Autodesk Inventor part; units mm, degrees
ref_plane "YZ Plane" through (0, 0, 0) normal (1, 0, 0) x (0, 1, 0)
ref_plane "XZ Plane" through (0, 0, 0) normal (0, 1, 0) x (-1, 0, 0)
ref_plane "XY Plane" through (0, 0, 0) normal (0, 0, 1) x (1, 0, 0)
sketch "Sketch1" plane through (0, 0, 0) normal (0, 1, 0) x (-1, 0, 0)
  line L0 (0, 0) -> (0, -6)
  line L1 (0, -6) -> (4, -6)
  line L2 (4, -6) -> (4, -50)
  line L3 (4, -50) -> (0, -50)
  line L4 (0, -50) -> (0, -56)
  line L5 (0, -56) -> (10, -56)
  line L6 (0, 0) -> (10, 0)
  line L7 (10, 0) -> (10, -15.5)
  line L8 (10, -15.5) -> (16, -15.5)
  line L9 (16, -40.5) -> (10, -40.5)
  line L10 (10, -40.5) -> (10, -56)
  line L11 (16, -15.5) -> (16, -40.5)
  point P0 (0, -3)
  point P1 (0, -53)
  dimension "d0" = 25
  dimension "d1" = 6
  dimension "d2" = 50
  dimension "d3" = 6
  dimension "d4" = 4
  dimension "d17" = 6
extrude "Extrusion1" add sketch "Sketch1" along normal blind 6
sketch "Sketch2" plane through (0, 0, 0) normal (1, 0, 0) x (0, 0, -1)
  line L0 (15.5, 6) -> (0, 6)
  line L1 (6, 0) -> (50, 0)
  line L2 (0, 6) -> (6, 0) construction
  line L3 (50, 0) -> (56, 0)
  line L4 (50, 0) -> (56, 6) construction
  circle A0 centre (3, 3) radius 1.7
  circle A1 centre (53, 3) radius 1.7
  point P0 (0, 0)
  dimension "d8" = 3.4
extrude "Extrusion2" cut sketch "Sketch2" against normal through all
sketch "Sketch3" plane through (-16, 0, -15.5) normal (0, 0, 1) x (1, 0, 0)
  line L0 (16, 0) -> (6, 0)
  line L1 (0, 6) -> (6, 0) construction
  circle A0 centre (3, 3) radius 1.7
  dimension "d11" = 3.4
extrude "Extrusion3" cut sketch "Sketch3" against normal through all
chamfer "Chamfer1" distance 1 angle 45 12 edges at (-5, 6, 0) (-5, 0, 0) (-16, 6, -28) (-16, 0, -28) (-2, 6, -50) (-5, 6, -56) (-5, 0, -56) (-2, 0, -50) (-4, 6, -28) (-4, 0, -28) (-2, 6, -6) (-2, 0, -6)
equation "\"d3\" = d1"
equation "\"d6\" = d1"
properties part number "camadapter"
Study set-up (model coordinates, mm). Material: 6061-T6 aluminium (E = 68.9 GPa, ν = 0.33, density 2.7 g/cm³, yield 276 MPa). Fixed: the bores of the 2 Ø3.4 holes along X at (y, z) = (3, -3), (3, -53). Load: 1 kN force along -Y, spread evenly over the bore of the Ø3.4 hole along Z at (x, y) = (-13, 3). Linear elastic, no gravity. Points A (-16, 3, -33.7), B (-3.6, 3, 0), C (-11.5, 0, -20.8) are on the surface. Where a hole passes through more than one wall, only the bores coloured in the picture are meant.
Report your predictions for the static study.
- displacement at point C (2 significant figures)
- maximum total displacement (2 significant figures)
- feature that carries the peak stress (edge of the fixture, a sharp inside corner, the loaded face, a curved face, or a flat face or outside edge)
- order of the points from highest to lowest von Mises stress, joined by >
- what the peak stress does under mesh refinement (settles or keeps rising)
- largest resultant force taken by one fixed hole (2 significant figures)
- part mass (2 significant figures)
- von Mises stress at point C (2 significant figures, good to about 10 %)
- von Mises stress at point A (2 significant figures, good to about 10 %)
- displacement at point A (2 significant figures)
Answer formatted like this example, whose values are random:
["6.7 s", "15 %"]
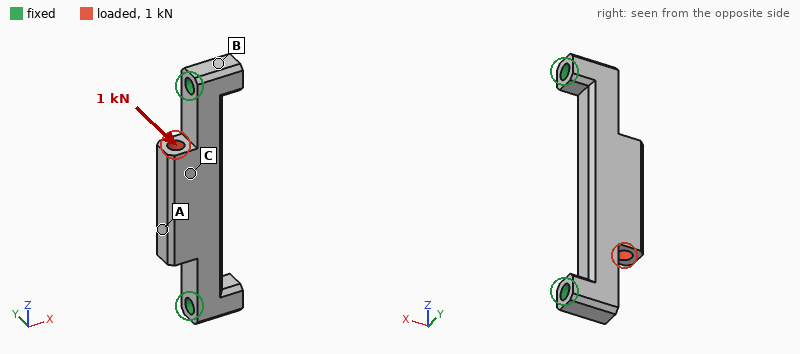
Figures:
["0.099 mm", "0.15 mm", "edge of the fixture", "C > A > B", "keeps rising", "500 N", "7.3 g", "60 MPa", "30 MPa", "0.14 mm"]
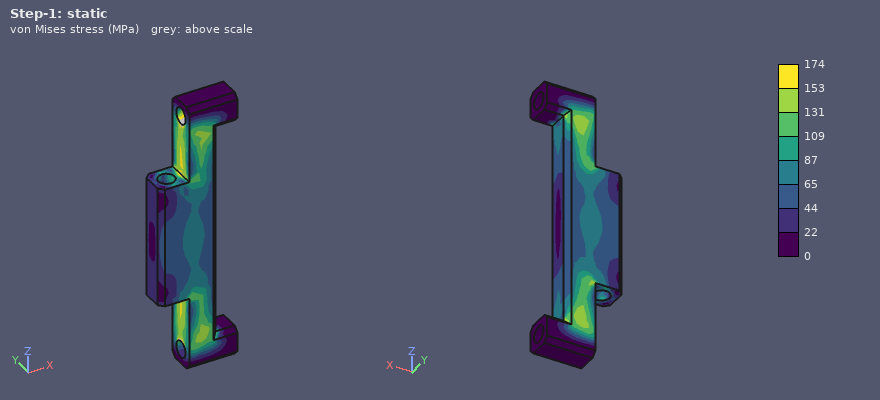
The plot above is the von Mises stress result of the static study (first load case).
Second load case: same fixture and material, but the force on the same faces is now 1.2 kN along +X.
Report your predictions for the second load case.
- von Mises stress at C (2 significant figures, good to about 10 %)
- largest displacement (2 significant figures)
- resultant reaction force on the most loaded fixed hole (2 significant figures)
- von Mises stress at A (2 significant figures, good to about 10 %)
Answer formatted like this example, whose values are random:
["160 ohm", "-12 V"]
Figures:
["36 MPa", "40 µm", "710 N", "31 MPa"]
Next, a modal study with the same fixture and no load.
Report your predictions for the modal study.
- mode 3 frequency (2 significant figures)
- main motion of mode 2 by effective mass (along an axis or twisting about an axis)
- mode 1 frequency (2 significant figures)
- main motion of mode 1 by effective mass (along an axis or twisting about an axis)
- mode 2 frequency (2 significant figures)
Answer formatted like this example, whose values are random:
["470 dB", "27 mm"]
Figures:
["18 kHz", "along X", "9100 Hz", "along Y", "14 kHz"]
